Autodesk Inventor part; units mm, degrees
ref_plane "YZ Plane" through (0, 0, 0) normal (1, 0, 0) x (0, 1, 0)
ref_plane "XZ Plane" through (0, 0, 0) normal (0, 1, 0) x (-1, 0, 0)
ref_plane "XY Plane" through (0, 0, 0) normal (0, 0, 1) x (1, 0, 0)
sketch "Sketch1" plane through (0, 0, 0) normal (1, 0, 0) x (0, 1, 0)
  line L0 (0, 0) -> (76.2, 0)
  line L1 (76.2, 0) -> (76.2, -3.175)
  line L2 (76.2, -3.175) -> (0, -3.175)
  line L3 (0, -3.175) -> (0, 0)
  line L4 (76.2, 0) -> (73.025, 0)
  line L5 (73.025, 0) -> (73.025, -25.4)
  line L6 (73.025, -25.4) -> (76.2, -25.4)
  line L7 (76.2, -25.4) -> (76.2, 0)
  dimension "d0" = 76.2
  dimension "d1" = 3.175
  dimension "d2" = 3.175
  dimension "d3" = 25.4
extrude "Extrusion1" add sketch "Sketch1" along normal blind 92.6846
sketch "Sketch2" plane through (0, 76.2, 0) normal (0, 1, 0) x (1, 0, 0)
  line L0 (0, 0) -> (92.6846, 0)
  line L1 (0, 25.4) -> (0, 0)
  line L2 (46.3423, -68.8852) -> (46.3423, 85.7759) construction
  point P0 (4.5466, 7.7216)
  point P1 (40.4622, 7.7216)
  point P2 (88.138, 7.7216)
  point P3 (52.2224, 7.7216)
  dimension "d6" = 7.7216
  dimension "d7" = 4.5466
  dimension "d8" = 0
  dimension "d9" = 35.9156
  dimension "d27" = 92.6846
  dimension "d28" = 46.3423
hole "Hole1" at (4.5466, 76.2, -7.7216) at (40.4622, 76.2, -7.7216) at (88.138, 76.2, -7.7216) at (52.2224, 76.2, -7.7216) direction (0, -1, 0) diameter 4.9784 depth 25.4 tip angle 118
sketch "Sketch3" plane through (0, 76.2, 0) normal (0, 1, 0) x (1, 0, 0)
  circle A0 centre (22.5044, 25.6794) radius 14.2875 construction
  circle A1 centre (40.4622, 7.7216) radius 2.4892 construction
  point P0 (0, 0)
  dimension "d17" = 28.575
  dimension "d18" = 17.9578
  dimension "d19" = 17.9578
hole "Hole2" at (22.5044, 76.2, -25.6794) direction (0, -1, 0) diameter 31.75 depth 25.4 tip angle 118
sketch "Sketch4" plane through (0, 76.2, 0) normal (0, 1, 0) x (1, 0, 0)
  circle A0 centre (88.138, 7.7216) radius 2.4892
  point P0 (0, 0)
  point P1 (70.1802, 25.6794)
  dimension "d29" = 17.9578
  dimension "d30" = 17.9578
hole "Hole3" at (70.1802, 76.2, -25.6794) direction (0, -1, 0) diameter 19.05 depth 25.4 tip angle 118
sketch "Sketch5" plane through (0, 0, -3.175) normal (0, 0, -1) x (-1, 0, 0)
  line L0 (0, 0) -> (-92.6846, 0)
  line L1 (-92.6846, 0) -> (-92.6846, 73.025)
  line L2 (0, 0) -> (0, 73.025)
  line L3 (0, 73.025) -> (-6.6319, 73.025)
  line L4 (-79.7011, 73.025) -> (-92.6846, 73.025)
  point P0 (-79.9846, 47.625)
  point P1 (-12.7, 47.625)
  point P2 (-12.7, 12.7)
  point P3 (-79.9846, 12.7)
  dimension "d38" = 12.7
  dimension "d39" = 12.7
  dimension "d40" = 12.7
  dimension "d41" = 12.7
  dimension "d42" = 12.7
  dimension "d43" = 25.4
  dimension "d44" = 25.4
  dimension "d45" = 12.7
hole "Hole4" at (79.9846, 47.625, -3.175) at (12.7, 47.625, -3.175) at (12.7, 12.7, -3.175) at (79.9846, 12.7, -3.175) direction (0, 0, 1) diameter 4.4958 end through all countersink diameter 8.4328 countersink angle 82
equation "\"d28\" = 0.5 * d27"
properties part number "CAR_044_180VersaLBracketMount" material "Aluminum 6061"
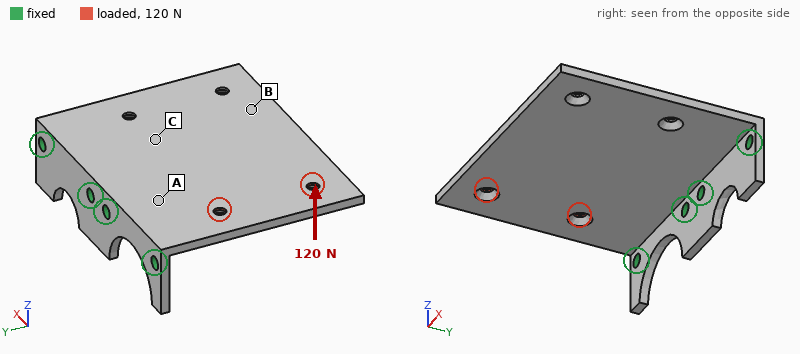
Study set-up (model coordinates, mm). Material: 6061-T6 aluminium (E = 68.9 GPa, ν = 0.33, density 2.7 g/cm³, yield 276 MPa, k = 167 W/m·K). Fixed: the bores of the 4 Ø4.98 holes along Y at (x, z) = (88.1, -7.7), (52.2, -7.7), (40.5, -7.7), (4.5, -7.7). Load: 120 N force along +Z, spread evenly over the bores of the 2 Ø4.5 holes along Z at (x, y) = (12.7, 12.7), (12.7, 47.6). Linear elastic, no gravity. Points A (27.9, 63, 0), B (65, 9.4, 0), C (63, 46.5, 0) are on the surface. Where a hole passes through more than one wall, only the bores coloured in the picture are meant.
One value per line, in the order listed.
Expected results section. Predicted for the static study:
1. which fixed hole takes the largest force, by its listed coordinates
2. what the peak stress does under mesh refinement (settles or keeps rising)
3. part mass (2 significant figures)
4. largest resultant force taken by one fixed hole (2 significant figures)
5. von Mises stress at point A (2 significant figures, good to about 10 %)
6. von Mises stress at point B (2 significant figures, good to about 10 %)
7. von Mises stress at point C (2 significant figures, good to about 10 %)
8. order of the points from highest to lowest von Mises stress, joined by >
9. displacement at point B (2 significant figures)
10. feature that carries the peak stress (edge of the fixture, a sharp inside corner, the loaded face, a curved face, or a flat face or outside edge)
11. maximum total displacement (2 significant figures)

(4.5, -7.7)
keeps rising
72 g
72 N
28 MPa
7.9 MPa
17 MPa
A > C > B
0.36 mm
edge of the fixture
0.77 mm
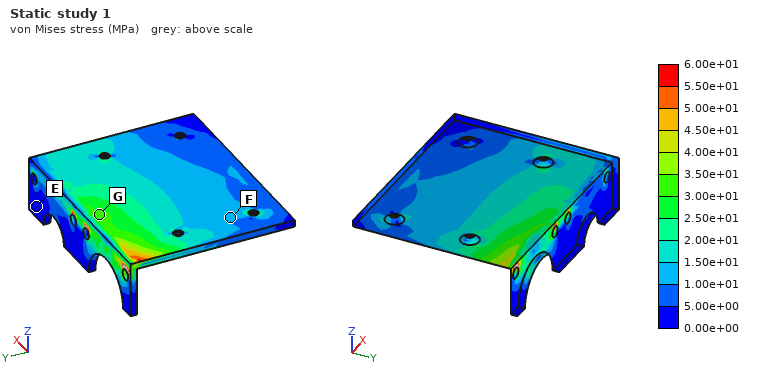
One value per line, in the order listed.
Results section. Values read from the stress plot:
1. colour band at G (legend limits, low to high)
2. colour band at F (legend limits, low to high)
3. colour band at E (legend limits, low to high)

3.00e+01 to 3.50e+01 MPa
1.00e+01 to 1.50e+01 MPa
0.00e+00 to 5.00e+00 MPa
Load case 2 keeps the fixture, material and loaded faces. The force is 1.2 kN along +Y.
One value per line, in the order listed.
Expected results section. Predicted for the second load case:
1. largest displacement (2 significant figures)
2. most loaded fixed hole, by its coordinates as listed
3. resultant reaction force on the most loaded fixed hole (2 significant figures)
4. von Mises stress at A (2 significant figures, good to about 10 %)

0.40 mm
(4.5, -7.7)
790 N
14 MPa
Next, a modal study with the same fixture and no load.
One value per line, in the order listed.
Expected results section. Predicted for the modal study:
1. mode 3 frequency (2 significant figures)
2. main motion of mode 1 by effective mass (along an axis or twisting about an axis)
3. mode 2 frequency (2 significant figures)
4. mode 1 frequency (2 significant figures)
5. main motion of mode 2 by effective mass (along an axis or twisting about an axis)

2400 Hz
along Z
930 Hz
430 Hz
twisting about Y
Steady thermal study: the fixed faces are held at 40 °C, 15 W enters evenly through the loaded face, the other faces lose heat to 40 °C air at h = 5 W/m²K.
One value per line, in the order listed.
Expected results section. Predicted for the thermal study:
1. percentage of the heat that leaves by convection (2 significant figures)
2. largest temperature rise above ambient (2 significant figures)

5.4 %
28 K
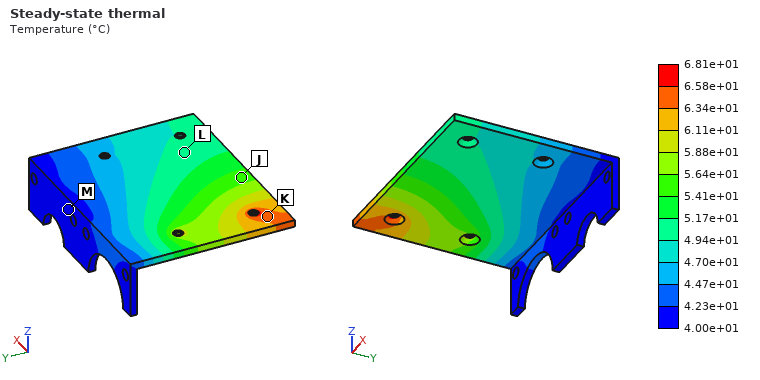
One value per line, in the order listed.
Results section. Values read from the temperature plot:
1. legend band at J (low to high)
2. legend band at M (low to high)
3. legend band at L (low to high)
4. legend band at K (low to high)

5.41e+01 to 5.64e+01 °C
4.00e+01 to 4.23e+01 °C
4.94e+01 to 5.17e+01 °C
6.34e+01 to 6.58e+01 °C
